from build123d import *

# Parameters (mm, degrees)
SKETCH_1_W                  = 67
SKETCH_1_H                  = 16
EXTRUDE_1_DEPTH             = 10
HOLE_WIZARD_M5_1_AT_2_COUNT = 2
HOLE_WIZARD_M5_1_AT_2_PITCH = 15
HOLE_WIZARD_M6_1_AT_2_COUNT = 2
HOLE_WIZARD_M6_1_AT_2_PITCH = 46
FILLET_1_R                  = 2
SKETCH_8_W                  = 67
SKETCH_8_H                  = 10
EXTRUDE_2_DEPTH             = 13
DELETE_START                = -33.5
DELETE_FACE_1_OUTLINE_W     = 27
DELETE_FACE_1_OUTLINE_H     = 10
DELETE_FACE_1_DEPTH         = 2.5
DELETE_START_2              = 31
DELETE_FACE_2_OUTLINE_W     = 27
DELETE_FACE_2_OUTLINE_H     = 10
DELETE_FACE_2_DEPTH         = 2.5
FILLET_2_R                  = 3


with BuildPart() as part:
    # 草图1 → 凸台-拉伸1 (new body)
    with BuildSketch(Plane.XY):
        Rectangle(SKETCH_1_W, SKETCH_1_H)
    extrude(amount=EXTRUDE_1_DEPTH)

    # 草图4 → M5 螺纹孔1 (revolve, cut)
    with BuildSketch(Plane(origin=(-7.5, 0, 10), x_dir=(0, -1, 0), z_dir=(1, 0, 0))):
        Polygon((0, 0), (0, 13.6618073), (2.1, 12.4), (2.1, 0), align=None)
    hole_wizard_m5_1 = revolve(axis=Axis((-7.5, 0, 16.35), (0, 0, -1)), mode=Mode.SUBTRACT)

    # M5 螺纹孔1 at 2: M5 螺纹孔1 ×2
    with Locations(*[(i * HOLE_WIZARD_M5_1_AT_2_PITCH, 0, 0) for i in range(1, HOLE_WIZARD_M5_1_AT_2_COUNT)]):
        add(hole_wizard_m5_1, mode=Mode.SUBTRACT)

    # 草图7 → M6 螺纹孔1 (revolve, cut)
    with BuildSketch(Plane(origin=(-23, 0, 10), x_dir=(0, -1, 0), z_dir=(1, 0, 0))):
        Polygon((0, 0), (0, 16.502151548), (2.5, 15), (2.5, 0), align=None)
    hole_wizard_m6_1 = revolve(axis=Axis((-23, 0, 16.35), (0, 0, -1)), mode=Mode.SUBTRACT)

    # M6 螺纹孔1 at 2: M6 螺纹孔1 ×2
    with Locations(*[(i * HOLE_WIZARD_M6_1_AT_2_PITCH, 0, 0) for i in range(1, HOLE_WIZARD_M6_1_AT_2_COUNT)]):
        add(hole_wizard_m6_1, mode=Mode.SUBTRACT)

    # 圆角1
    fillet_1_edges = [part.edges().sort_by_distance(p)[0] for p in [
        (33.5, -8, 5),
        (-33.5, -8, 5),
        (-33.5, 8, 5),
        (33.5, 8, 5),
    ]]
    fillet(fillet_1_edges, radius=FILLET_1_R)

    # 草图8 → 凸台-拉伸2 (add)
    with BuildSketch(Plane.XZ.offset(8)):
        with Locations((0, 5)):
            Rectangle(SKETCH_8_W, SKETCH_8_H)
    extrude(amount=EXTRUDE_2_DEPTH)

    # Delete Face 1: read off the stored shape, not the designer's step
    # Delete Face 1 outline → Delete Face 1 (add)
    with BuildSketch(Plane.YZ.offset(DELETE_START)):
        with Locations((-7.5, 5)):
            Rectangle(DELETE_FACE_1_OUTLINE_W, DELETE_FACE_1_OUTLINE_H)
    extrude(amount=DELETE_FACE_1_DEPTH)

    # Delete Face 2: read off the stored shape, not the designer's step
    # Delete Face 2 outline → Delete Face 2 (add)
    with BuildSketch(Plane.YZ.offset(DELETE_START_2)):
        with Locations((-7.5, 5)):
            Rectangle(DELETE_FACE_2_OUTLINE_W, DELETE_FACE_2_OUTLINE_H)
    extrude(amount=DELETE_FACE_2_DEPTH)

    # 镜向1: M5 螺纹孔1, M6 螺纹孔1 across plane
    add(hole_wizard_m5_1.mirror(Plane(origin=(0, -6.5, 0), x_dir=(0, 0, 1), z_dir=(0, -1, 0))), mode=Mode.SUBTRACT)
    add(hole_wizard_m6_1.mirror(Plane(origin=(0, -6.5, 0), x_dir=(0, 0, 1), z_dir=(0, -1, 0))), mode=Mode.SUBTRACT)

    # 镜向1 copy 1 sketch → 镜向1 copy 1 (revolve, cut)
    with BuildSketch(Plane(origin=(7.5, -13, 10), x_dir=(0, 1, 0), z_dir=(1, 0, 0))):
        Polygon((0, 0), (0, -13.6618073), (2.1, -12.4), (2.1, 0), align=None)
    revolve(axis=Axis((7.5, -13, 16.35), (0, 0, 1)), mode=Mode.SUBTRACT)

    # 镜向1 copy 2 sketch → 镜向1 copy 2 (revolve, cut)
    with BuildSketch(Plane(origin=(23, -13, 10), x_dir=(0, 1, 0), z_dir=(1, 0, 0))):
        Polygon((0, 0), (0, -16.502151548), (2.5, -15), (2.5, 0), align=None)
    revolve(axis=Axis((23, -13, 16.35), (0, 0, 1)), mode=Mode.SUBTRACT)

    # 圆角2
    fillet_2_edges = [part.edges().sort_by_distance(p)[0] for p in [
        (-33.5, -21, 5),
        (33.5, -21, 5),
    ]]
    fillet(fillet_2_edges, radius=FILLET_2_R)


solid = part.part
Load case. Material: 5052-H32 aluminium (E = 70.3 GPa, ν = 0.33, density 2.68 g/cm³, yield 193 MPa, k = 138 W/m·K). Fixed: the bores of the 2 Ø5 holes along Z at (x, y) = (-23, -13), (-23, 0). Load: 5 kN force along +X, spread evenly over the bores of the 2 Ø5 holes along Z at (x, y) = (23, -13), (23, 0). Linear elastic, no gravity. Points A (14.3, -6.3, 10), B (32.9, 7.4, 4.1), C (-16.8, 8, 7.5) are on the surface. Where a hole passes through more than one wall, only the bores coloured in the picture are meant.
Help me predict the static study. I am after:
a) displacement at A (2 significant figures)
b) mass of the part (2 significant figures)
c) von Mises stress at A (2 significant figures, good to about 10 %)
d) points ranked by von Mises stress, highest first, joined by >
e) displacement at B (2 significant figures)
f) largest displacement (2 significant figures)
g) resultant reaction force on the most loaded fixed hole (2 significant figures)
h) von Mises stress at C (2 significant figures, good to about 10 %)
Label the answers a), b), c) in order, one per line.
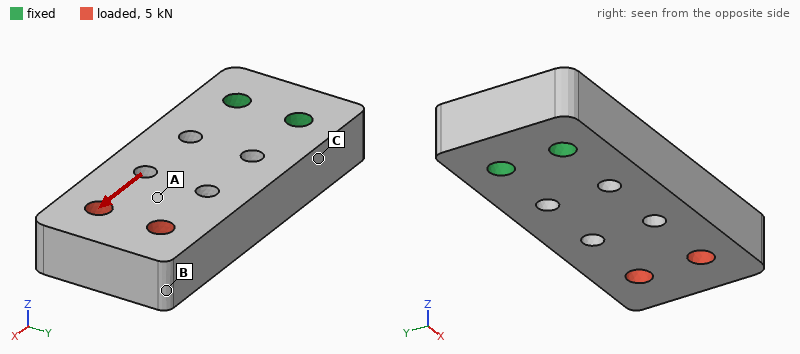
a) 11 µm
b) 48 g
c) 23 MPa
d) A > C > B
e) 12 µm
f) 15 µm
g) 2.5 kN
h) 13 MPa
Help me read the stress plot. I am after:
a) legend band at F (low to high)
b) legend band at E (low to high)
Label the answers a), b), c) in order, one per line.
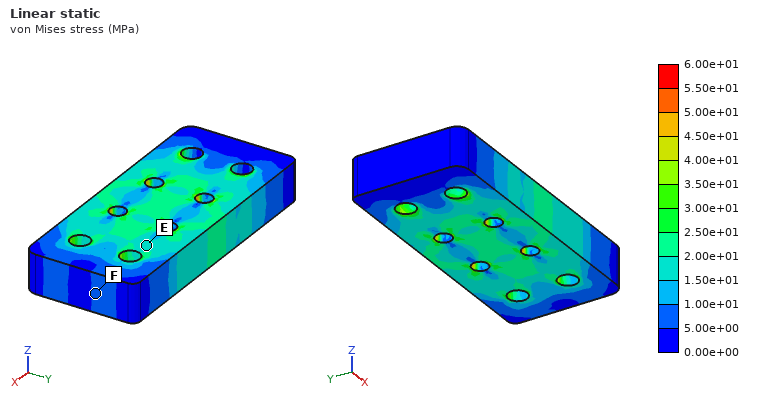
a) 5.00e+00 to 1.00e+01 MPa
b) 1.50e+01 to 2.00e+01 MPa
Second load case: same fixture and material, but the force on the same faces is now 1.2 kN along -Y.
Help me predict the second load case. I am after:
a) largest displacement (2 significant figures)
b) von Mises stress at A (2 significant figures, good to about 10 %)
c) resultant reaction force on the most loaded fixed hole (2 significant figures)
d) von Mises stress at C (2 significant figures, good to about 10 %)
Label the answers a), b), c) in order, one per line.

a) 58 µm
b) 7.9 MPa
c) 3.3 kN
d) 29 MPa
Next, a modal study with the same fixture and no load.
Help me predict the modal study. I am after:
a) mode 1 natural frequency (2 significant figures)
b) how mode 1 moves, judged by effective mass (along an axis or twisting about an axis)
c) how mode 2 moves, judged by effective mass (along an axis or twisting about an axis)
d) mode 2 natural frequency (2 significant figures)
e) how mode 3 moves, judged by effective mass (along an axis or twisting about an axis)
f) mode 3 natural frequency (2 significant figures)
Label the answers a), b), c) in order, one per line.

a) 2600 Hz
b) along Z
c) along Y
d) 5900 Hz
e) twisting about X
f) 8500 Hz
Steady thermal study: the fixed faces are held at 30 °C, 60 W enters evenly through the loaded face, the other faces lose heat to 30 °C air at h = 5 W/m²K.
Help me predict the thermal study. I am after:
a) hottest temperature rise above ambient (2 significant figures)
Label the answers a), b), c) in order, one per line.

a) 78 K
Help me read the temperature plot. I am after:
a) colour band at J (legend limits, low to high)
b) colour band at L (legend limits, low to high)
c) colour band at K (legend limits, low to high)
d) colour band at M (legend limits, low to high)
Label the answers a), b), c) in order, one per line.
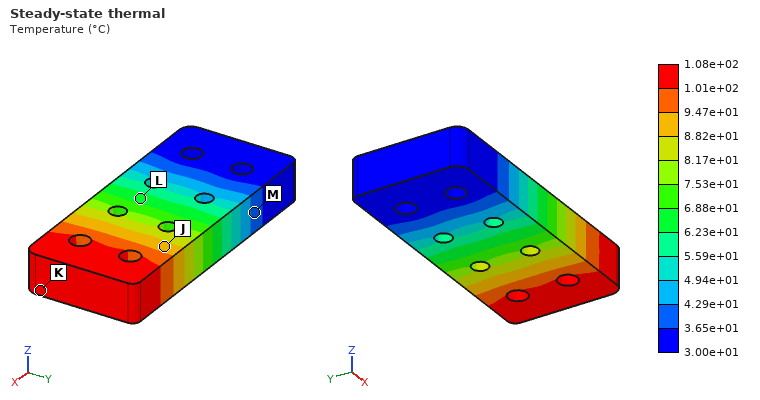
a) 8.82e+01 to 9.47e+01 °C
b) 6.23e+01 to 6.88e+01 °C
c) 1.01e+02 to 1.08e+02 °C
d) 3.65e+01 to 4.29e+01 °C
